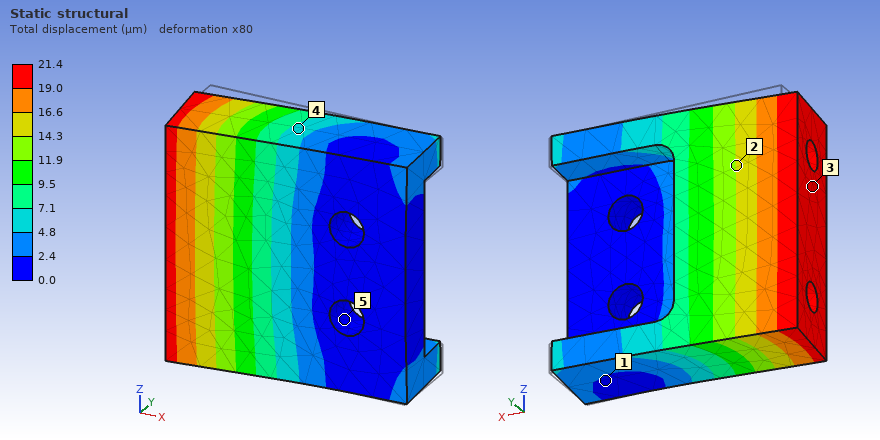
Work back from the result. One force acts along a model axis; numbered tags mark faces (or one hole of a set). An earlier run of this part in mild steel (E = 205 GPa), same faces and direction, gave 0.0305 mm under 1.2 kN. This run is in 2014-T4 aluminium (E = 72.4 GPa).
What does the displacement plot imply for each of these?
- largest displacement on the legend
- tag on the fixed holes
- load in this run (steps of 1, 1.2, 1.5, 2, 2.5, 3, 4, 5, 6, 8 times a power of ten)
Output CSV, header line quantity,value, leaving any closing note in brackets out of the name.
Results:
quantity,value
largest displacement on the legend,21.4 µm
tag on the fixed holes,5
load in this run,300 N
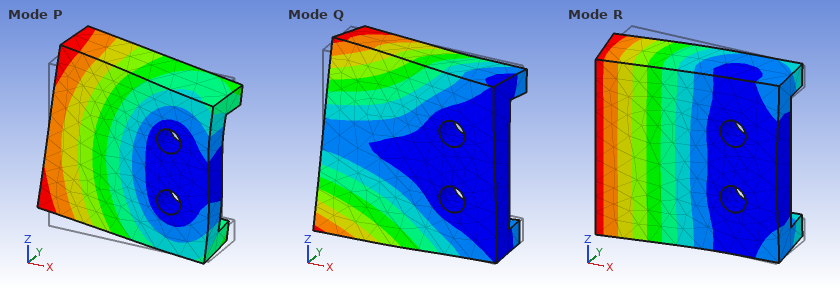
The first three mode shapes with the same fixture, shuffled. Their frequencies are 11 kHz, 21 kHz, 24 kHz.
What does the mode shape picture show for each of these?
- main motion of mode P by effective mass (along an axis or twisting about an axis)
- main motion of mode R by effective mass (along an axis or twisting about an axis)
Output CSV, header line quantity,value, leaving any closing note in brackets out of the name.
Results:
quantity,value
main motion of mode P by effective mass,along Z
main motion of mode R by effective mass,along Y
